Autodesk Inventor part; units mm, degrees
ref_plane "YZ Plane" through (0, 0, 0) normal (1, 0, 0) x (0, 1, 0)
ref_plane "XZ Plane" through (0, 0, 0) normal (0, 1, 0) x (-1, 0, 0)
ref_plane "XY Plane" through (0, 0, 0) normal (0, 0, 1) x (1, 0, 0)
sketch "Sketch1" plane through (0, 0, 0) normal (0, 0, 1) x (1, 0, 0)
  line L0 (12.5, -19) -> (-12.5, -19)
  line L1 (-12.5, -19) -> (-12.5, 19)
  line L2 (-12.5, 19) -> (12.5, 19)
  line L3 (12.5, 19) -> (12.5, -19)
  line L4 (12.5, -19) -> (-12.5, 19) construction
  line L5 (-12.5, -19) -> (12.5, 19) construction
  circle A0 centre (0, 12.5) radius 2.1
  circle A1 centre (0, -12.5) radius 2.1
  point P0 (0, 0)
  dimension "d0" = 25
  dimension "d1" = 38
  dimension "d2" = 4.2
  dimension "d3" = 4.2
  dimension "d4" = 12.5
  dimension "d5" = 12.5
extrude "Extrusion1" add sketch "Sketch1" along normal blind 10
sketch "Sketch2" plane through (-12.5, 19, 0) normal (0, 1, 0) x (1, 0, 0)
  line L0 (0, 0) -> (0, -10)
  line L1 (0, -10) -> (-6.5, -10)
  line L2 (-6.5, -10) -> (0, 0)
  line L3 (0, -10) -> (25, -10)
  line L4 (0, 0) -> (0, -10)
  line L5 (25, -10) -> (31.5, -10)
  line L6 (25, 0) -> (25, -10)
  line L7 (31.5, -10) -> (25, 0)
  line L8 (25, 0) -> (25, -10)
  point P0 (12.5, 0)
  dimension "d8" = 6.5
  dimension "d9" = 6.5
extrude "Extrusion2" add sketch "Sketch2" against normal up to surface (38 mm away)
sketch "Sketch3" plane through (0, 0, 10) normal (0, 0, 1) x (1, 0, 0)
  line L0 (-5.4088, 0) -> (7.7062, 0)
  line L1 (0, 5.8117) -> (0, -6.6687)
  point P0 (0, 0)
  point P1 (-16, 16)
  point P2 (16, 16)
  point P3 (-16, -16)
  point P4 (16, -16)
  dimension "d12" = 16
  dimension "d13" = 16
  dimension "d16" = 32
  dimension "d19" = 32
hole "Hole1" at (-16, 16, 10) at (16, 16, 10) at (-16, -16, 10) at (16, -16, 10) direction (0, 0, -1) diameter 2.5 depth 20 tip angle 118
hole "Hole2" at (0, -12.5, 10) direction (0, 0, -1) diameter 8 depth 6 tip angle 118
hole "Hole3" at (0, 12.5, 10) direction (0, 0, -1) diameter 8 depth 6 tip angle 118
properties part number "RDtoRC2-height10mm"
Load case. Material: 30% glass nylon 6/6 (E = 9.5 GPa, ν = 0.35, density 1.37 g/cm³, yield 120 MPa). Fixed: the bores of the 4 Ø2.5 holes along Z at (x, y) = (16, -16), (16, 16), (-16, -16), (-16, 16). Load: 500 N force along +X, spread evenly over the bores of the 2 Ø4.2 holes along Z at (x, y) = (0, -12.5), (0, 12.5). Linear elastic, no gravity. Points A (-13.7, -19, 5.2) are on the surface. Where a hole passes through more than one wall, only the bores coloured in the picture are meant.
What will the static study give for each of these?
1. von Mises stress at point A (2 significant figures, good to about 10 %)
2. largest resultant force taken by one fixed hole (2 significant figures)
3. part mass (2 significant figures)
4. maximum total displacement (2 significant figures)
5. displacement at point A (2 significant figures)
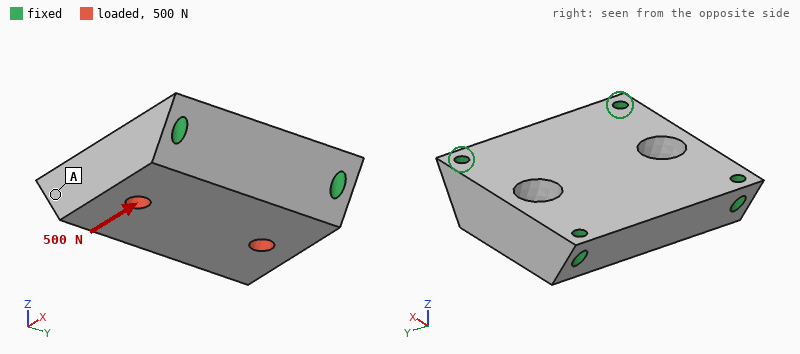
1.1 MPa
140 N
15 g
6.2 µm
1.00 µm
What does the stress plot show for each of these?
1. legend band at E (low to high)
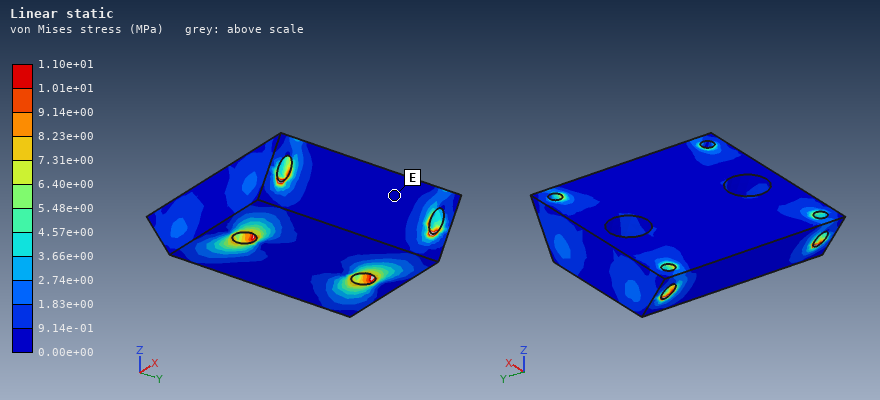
0.00e+00 to 9.14e-01 MPa
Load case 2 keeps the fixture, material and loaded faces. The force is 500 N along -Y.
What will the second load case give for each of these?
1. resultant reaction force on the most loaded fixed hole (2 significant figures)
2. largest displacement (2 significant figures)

150 N
12 µm
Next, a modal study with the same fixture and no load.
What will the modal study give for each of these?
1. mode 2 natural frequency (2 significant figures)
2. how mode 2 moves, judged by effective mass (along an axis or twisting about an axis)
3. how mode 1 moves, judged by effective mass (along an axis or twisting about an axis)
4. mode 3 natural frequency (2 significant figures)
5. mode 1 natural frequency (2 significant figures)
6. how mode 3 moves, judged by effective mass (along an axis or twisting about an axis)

14 kHz
along X
along Z
16 kHz
9600 Hz
along Y
